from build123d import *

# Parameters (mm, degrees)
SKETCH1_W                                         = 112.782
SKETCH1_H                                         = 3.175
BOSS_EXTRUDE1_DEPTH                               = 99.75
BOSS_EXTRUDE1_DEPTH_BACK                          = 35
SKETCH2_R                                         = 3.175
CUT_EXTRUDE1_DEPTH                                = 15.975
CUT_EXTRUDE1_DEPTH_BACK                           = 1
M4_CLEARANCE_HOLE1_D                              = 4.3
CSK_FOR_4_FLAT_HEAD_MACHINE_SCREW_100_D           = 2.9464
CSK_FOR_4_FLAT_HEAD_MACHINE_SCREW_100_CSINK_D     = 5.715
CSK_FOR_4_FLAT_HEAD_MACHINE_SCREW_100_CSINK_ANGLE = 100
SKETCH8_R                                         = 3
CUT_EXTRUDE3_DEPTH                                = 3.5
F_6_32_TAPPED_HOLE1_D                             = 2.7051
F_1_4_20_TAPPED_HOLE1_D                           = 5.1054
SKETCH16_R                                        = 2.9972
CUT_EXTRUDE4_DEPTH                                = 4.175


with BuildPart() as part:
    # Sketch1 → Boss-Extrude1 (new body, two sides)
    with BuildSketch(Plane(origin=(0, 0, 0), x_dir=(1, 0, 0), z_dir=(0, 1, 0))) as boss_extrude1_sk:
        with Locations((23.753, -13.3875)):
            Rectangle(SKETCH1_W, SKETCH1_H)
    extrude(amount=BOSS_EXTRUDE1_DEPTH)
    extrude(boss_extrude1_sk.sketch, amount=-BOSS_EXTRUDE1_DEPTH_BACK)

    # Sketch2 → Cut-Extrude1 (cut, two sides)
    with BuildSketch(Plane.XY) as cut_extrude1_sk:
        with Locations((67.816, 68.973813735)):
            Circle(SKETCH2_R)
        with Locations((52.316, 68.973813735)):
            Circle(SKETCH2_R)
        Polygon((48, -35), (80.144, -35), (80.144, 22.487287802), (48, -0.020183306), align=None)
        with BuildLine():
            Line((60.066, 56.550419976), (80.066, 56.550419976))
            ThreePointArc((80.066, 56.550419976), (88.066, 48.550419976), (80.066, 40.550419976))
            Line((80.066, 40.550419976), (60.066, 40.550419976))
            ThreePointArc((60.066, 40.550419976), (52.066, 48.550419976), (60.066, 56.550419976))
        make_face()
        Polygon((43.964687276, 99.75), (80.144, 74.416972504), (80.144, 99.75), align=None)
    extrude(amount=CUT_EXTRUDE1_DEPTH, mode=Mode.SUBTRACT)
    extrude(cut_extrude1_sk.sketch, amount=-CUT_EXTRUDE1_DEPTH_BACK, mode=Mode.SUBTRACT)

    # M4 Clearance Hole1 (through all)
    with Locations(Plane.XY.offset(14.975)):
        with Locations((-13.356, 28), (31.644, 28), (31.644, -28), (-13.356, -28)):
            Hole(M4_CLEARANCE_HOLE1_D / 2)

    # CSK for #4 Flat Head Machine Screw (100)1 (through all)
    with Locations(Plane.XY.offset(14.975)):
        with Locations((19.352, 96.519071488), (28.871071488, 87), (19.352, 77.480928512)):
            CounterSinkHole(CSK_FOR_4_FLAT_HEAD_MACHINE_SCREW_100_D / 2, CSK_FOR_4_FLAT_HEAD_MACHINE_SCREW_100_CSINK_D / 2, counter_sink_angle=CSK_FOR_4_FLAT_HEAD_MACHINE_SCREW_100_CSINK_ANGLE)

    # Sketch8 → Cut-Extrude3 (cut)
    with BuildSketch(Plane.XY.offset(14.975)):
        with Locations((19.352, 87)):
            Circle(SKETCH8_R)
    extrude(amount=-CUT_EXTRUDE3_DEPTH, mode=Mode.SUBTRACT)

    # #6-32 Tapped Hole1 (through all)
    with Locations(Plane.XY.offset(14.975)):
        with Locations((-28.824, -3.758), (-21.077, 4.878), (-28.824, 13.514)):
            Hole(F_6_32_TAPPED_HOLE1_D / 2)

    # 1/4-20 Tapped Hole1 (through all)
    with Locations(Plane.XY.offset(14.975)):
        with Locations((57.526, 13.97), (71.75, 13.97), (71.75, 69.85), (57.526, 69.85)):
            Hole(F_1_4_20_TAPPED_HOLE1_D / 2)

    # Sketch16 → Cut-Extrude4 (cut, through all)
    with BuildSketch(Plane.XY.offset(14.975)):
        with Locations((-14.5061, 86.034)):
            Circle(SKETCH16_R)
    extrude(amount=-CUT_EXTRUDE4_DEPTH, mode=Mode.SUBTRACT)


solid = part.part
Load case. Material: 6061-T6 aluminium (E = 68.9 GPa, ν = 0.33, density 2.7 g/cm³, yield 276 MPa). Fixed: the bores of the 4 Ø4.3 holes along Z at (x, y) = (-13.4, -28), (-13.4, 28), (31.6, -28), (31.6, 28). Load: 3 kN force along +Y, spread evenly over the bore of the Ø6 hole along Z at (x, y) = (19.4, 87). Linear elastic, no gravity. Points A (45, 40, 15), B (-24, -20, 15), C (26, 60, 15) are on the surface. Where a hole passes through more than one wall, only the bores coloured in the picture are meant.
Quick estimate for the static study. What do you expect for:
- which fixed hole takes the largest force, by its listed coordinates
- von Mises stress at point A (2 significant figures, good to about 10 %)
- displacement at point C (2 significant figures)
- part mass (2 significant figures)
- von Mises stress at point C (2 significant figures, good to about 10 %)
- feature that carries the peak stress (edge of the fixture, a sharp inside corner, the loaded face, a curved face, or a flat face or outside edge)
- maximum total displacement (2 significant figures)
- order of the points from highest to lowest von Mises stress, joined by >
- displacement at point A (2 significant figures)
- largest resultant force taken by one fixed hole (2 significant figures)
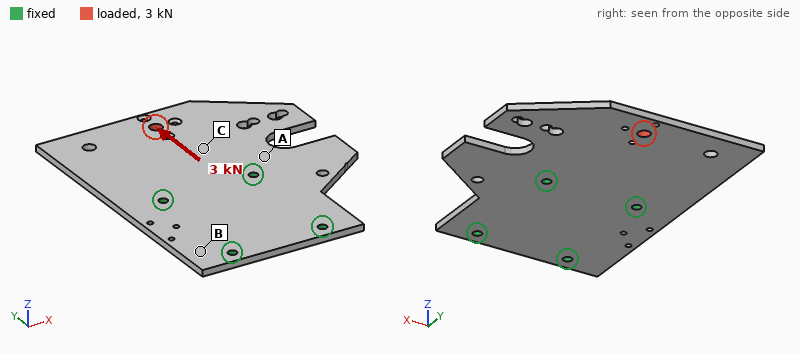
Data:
(31.6, 28)
11 MPa
11 µm
110 g
21 MPa
a curved face
28 µm
C > A > B
7.1 µm
1.7 kN
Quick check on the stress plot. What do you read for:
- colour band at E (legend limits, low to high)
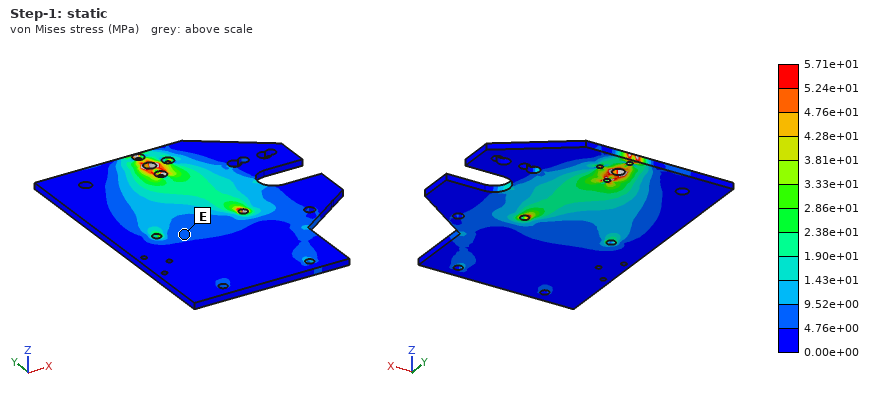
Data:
4.76e+00 to 9.52e+00 MPa
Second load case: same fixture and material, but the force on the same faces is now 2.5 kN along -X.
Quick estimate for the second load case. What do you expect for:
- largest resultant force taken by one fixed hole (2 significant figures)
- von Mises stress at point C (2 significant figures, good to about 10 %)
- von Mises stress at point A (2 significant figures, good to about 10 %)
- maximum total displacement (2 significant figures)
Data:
2.6 kN
22 MPa
17 MPa
67 µm
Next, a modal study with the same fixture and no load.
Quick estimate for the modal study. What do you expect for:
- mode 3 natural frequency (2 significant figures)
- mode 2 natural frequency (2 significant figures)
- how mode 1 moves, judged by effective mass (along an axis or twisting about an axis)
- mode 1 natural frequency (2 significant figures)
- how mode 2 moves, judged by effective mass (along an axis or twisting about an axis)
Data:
1500 Hz
810 Hz
along Z
480 Hz
twisting about Y
